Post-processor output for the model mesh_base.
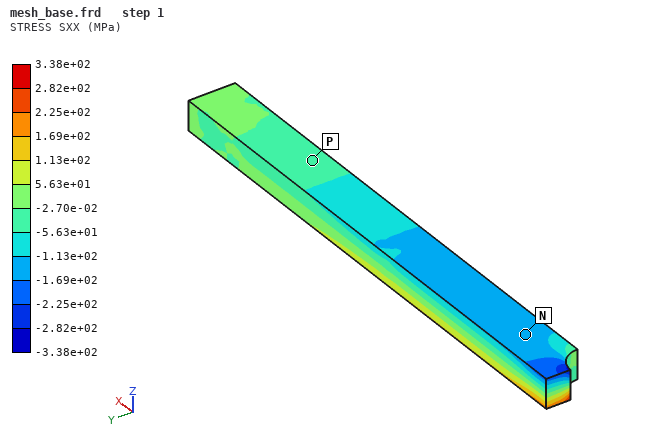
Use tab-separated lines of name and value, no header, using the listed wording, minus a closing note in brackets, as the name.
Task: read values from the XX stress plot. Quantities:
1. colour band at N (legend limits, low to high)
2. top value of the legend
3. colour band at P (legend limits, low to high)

colour band at N	-1.69e+02 to -1.13e+02 MPa
top value of the legend	3.38e+02 MPa
colour band at P	-5.63e+01 to -2.70e-02 MPa
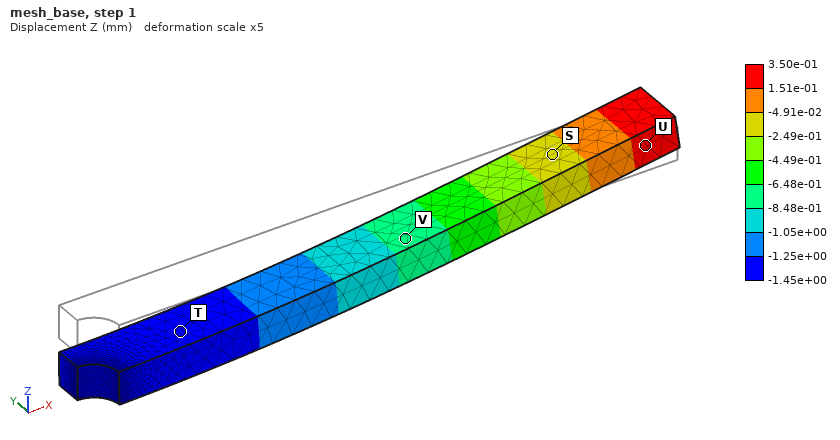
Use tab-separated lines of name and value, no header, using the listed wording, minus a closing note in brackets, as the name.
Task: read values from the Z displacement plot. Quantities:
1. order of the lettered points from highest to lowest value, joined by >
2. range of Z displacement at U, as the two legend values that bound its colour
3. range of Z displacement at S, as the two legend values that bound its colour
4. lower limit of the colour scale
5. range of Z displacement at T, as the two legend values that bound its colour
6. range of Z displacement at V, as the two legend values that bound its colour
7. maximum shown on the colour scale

order of the lettered points from highest to lowest value, joined by >	U > S > V > T
range of Z displacement at U, as the two legend values that bound its colour	1.51e-01 to 3.50e-01 mm
range of Z displacement at S, as the two legend values that bound its colour	-2.49e-01 to -4.91e-02 mm
lower limit of the colour scale	-1.45e+00 mm
range of Z displacement at T, as the two legend values that bound its colour	-1.45e+00 to -1.25e+00 mm
range of Z displacement at V, as the two legend values that bound its colour	-8.48e-01 to -6.48e-01 mm
maximum shown on the colour scale	3.50e-01 mm
